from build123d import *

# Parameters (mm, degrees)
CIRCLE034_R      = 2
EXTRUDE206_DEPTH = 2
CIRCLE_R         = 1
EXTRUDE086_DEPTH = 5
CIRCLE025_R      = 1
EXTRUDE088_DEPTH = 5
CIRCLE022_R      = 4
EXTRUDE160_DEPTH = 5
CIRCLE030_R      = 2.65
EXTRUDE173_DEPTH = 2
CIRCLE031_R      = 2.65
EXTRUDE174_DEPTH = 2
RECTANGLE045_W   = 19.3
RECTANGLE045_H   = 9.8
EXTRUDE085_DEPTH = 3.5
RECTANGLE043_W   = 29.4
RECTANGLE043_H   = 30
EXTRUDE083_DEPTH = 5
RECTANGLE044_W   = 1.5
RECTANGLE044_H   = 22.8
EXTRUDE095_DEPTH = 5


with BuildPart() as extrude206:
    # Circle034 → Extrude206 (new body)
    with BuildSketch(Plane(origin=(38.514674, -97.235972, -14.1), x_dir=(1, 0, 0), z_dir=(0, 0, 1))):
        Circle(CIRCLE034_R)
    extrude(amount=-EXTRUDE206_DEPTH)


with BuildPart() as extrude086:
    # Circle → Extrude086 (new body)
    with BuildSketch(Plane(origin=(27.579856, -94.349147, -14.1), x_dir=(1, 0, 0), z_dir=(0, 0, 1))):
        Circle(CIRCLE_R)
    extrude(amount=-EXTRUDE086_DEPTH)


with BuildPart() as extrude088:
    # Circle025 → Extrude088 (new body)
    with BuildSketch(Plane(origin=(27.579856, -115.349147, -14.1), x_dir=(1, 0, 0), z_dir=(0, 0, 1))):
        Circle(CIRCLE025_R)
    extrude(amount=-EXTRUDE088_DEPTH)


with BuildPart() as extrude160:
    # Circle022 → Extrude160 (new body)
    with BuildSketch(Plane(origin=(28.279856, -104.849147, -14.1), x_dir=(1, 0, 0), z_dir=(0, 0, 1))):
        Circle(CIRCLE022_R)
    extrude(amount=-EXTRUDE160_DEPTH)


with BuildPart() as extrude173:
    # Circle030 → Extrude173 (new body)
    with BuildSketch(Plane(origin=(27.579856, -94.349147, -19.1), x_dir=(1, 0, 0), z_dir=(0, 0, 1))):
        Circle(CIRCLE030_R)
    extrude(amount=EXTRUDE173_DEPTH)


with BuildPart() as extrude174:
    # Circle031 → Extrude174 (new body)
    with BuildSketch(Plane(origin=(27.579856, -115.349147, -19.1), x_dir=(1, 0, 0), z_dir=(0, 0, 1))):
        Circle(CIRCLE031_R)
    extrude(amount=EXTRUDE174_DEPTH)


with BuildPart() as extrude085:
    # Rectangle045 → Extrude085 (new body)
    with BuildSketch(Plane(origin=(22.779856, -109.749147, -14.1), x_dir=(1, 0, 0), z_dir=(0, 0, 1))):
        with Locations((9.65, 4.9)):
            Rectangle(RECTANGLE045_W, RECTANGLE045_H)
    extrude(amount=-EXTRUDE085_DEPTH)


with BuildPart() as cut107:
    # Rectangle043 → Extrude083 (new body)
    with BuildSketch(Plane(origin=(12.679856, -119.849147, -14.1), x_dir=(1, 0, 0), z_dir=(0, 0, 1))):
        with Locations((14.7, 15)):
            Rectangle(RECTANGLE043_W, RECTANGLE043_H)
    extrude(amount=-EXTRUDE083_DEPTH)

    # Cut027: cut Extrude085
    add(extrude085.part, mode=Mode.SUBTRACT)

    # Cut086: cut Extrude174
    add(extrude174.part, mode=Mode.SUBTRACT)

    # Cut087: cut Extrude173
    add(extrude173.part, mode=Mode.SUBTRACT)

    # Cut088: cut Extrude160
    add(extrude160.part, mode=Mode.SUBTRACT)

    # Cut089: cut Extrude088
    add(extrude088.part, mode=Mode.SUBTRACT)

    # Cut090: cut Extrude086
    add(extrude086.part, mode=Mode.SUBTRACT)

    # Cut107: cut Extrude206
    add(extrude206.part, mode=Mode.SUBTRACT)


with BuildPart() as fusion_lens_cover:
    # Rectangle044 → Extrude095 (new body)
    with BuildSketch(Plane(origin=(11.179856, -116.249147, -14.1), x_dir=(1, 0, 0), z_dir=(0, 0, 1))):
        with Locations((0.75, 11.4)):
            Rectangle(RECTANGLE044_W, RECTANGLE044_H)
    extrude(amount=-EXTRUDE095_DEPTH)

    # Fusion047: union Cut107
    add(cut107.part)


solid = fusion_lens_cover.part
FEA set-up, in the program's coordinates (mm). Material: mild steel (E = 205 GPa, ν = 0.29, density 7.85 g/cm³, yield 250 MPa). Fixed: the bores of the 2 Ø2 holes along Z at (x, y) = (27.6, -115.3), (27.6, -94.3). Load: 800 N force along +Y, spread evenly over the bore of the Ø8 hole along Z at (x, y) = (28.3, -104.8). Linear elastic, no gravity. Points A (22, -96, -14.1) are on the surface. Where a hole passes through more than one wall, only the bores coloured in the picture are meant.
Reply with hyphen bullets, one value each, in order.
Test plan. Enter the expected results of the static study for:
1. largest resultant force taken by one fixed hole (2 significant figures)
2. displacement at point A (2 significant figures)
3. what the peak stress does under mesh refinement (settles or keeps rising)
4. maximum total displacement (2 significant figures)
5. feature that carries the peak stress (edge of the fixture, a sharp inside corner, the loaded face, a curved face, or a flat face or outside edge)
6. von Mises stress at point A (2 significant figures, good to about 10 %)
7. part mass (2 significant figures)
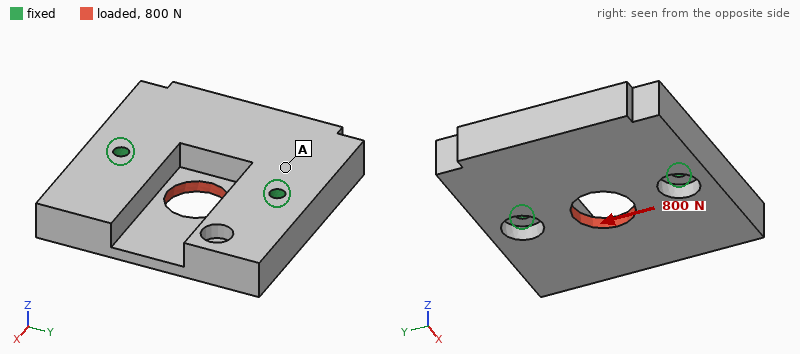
- 410 N
- 0.30 µm
- keeps rising
- 2.0 µm
- edge of the fixture
- 6.5 MPa
- 29 g
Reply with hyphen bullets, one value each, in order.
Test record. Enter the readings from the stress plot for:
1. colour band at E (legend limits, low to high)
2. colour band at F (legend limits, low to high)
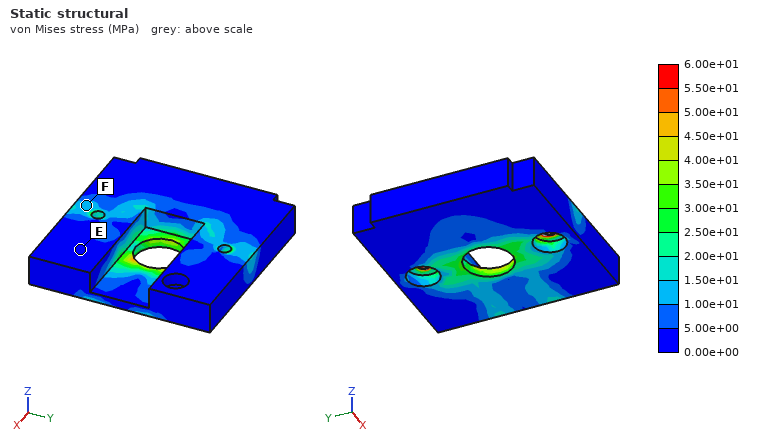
- 0.00e+00 to 5.00e+00 MPa
- 1.00e+01 to 1.50e+01 MPa
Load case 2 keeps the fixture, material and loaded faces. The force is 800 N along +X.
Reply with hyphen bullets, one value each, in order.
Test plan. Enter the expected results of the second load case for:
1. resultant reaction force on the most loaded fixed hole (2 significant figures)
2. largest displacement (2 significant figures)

- 400 N
- 7.7 µm
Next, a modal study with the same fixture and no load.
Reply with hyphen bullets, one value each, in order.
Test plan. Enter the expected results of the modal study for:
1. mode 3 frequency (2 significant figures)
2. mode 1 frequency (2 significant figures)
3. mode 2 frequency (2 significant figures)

- 14 kHz
- 7100 Hz
- 14 kHz
